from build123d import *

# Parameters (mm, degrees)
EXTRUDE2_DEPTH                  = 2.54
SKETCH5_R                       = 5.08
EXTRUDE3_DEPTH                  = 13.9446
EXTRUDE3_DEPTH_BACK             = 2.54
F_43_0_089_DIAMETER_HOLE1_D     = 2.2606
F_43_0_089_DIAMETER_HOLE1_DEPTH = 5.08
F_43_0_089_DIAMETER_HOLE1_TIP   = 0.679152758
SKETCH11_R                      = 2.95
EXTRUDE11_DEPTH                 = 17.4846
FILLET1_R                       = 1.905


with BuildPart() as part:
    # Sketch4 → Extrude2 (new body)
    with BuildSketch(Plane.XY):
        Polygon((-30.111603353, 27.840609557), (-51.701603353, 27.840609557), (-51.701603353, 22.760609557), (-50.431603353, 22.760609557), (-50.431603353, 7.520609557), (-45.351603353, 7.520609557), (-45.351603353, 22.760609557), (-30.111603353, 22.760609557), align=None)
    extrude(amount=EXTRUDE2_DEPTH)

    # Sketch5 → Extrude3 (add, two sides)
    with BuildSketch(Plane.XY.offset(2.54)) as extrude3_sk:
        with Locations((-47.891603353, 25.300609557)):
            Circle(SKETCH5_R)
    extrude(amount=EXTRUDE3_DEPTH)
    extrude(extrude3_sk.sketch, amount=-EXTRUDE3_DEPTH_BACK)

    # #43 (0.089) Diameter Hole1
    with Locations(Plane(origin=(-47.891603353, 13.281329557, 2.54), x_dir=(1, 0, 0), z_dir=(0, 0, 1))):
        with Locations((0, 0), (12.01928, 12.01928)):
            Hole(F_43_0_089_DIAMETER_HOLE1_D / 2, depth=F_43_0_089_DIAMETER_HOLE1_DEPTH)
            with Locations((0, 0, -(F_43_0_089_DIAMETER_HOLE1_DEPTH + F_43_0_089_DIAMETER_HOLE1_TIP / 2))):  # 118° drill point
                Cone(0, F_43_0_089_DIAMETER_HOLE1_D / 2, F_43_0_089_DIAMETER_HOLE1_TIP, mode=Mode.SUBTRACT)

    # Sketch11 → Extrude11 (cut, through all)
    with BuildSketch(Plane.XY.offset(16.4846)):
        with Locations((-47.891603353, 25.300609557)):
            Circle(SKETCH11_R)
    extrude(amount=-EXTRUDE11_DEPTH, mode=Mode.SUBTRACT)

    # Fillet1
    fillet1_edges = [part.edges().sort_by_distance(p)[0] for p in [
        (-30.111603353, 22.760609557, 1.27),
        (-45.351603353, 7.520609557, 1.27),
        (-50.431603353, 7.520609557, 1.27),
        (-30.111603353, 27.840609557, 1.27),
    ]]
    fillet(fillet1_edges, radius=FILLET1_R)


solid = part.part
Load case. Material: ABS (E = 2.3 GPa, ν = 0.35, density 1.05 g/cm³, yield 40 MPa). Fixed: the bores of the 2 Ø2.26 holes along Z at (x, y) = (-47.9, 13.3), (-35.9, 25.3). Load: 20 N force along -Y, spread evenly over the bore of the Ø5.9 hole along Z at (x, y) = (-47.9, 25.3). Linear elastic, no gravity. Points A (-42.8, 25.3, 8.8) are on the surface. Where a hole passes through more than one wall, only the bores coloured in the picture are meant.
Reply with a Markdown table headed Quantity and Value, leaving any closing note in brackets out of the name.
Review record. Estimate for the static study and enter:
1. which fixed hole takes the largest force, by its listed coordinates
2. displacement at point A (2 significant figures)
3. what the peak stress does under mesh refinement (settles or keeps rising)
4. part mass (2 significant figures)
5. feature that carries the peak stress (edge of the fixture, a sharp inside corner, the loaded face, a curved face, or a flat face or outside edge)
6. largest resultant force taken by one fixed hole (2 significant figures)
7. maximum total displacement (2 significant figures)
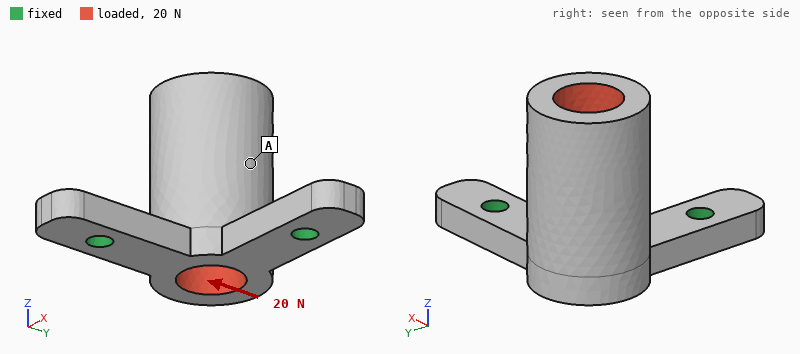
| Quantity | Value |
|---|---|
| which fixed hole takes the largest force, by its listed coordinates | (-47.9, 13.3) |
| displacement at point A | 0.19 mm |
| what the peak stress does under mesh refinement | keeps rising |
| part mass | 1.3 g |
| feature that carries the peak stress | edge of the fixture |
| largest resultant force taken by one fixed hole | 21 N |
| maximum total displacement | 0.43 mm |
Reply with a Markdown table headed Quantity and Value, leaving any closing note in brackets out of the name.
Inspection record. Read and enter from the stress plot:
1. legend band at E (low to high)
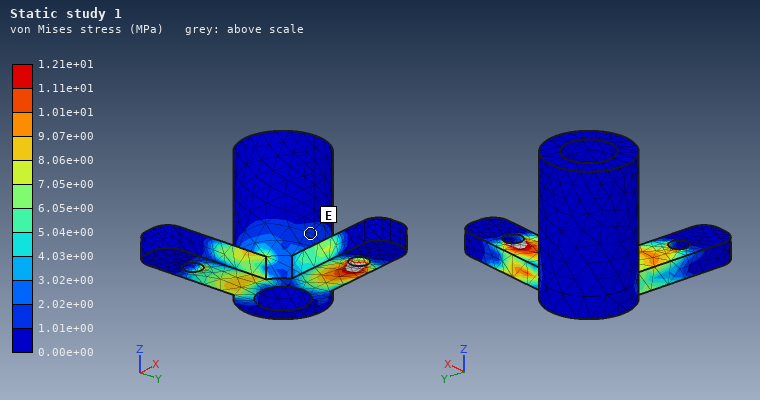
| Quantity | Value |
|---|---|
| legend band at E | 1.01e+00 to 2.02e+00 MPa |
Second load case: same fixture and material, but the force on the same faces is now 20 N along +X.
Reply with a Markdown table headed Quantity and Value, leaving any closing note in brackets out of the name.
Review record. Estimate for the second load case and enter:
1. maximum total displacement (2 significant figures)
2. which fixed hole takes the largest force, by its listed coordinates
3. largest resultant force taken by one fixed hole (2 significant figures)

| Quantity | Value |
|---|---|
| maximum total displacement | 0.43 mm |
| which fixed hole takes the largest force, by its listed coordinates | (-35.9, 25.3) |
| largest resultant force taken by one fixed hole | 21 N |
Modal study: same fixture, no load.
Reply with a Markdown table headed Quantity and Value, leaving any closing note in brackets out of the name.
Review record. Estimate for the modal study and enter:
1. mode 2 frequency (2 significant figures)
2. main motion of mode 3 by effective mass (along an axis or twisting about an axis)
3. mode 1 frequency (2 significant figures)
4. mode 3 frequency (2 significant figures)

| Quantity | Value |
|---|---|
| mode 2 frequency | 2500 Hz |
| main motion of mode 3 by effective mass | along Z |
| mode 1 frequency | 1000 Hz |
| mode 3 frequency | 4500 Hz |
